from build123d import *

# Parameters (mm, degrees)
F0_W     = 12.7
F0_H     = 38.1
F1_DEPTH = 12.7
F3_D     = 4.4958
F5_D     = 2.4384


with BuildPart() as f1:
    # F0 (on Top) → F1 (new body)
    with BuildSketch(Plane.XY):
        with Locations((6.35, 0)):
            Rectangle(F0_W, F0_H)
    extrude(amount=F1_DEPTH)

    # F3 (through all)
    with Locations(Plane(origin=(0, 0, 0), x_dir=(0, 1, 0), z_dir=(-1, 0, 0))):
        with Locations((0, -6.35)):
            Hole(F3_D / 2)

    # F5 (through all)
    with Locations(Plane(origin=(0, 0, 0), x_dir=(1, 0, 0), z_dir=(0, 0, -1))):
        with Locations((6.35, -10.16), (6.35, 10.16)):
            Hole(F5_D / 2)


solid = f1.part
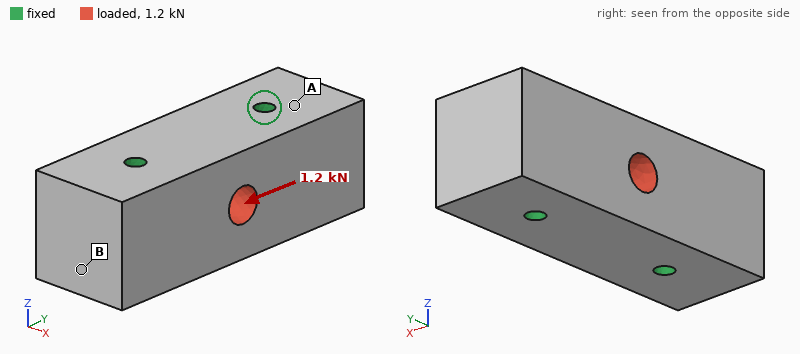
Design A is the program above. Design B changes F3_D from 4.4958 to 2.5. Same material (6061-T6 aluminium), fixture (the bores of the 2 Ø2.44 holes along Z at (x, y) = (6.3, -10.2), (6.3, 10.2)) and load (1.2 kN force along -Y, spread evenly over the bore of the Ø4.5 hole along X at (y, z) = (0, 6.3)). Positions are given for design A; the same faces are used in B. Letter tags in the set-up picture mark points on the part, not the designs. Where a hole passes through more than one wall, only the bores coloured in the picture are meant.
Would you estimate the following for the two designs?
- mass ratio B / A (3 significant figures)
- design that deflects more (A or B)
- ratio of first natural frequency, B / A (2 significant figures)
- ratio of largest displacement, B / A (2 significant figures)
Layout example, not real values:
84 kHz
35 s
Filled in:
1.02
B
1.0
1.2
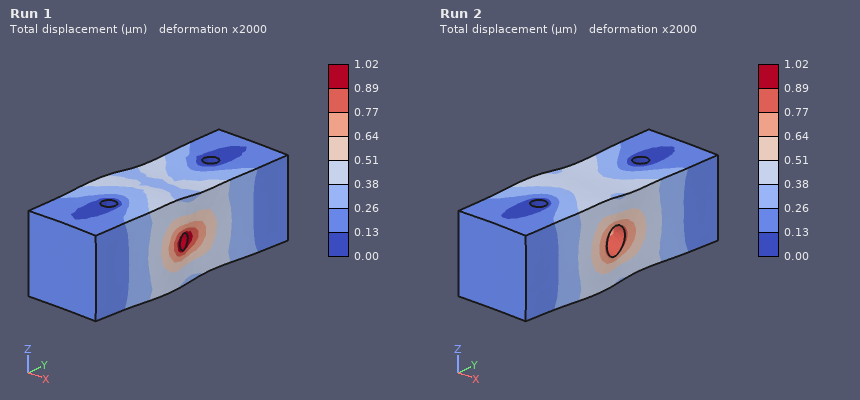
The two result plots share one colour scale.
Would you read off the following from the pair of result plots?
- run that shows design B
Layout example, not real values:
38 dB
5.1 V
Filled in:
Run 1
